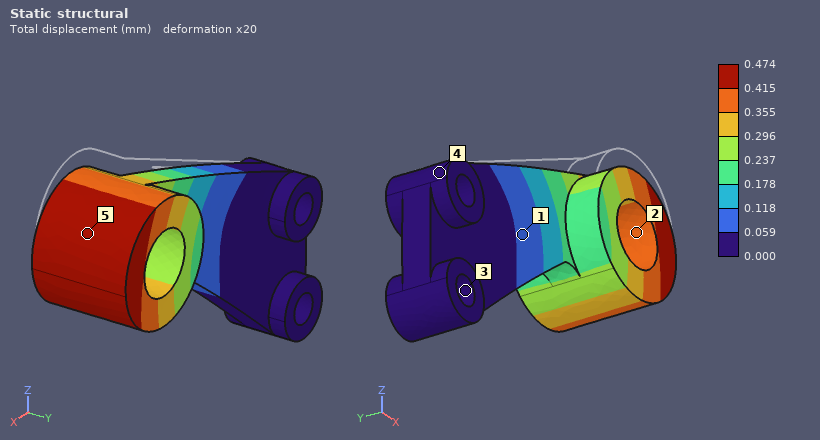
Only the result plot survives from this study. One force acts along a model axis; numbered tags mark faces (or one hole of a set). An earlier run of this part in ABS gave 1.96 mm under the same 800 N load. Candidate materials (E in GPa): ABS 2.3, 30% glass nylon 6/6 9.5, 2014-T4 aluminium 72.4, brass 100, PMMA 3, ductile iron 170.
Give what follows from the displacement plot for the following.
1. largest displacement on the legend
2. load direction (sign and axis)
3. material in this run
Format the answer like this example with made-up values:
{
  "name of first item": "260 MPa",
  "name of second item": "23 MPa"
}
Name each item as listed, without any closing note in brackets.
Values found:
{
  "largest displacement on the legend": "0.474 mm",
  "load direction": "-Z",
  "material in this run": "30% glass nylon 6/6"
}
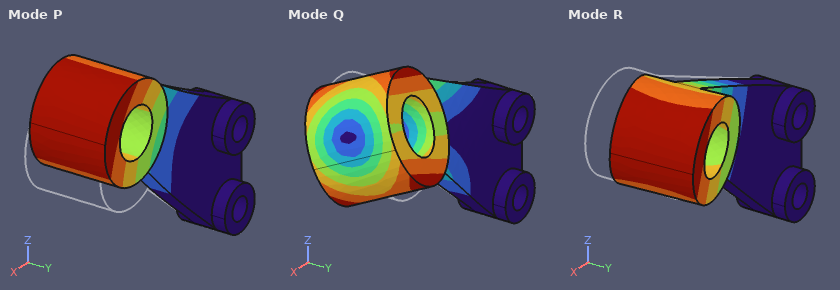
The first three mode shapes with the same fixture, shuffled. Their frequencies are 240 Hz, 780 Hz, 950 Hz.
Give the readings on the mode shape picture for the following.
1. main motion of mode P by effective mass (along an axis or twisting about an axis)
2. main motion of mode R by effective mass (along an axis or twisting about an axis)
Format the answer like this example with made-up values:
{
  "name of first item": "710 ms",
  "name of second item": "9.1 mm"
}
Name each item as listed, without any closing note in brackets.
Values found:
{
  "main motion of mode P by effective mass": "along Z",
  "main motion of mode R by effective mass": "along Y"
}
